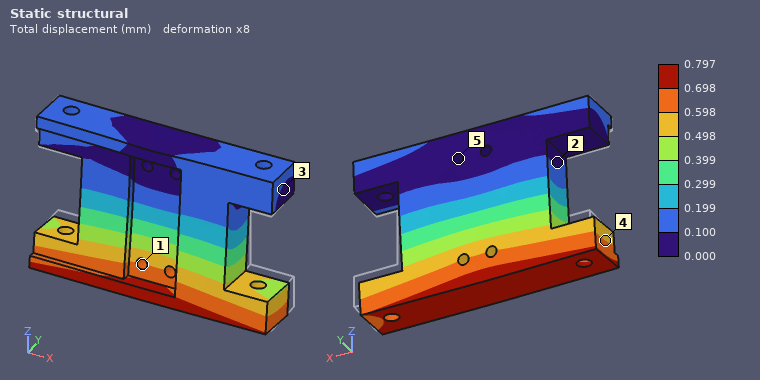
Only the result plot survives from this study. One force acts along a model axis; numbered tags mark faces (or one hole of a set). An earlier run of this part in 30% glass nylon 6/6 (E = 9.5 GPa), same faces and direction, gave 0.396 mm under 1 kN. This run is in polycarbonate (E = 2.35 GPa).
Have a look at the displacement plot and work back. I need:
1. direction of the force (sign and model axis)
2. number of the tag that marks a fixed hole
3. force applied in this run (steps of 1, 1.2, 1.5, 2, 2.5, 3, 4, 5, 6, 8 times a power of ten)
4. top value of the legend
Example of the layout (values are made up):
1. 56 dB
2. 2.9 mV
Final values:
1. -Y
2. 5
3. 500 N
4. 0.797 mm
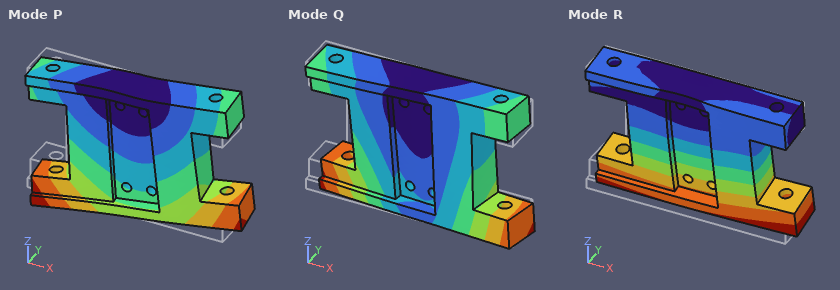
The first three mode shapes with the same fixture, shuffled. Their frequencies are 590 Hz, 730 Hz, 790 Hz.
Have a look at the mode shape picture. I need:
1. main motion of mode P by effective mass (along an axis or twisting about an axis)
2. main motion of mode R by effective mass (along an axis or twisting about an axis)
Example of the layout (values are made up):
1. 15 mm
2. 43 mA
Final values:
1. along X
2. along Y
